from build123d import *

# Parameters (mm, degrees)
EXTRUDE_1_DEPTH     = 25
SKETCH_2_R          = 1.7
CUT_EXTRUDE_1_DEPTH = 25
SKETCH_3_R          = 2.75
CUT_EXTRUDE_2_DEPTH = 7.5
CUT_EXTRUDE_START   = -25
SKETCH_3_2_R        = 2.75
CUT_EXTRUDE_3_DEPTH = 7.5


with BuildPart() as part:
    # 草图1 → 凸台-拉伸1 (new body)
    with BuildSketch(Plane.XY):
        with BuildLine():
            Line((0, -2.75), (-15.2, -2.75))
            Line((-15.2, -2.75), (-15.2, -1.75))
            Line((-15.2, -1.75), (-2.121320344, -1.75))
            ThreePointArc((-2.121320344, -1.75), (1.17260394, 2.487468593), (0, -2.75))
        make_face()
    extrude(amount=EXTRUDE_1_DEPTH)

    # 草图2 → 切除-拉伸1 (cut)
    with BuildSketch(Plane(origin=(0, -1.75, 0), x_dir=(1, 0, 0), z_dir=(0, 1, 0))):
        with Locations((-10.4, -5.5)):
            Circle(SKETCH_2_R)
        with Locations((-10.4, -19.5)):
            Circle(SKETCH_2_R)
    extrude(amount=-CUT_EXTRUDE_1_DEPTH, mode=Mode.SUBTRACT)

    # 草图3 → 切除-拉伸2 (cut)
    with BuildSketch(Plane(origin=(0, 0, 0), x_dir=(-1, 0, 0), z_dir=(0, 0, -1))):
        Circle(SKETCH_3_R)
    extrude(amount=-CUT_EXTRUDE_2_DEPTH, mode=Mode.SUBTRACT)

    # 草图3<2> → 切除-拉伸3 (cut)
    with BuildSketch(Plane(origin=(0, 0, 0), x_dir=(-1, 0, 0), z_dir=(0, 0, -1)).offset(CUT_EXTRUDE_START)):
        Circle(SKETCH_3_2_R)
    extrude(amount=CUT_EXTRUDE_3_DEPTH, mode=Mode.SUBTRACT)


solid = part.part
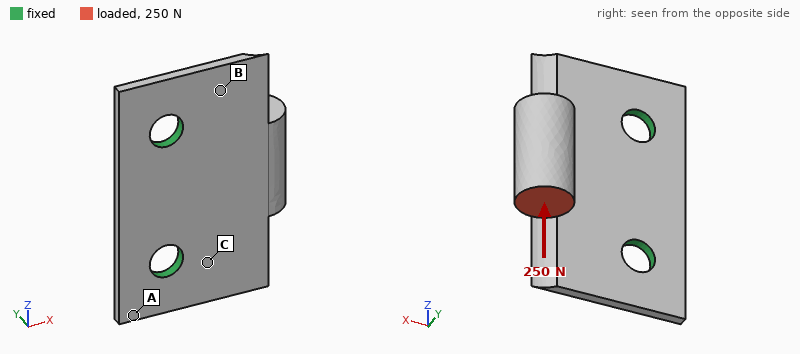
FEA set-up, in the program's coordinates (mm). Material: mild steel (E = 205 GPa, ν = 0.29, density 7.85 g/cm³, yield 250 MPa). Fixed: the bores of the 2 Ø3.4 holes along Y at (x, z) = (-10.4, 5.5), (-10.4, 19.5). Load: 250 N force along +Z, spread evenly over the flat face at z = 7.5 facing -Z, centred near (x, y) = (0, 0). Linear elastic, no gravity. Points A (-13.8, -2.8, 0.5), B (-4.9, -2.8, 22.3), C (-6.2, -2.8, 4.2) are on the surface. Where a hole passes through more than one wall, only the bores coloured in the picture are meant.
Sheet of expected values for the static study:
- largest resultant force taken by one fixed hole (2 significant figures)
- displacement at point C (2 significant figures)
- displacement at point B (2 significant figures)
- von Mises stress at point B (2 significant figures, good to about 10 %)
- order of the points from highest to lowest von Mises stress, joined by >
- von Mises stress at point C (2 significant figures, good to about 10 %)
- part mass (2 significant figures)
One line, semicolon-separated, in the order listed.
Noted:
200 N; 4.5 µm; 7.7 µm; 34 MPa; C > B > A; 63 MPa; 4.4 g
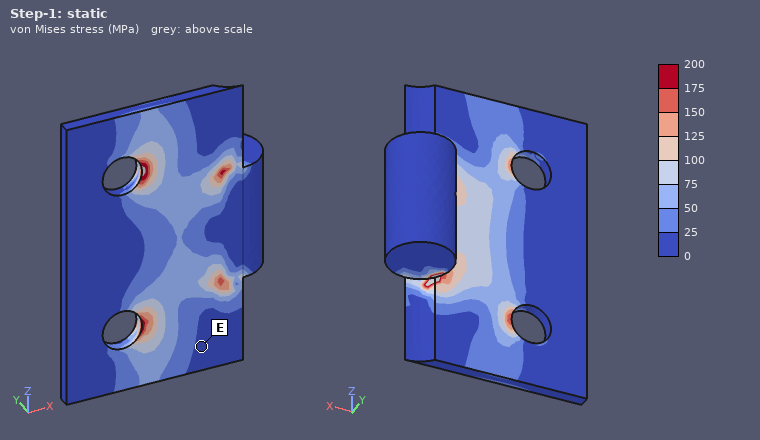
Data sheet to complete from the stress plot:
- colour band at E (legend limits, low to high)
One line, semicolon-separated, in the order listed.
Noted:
0 to 25 MPa
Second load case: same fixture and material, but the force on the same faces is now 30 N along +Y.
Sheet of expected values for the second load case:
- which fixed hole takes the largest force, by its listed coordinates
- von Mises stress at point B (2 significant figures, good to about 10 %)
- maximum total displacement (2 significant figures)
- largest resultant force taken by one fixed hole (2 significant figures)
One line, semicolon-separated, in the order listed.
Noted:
(-10.4, 5.5); 27 MPa; 39 µm; 27 N
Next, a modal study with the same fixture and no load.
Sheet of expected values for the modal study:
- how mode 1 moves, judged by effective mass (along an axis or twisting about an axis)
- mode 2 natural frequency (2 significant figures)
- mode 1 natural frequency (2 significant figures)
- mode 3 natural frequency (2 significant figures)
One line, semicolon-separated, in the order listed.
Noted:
along Y; 11 kHz; 3600 Hz; 15 kHz
